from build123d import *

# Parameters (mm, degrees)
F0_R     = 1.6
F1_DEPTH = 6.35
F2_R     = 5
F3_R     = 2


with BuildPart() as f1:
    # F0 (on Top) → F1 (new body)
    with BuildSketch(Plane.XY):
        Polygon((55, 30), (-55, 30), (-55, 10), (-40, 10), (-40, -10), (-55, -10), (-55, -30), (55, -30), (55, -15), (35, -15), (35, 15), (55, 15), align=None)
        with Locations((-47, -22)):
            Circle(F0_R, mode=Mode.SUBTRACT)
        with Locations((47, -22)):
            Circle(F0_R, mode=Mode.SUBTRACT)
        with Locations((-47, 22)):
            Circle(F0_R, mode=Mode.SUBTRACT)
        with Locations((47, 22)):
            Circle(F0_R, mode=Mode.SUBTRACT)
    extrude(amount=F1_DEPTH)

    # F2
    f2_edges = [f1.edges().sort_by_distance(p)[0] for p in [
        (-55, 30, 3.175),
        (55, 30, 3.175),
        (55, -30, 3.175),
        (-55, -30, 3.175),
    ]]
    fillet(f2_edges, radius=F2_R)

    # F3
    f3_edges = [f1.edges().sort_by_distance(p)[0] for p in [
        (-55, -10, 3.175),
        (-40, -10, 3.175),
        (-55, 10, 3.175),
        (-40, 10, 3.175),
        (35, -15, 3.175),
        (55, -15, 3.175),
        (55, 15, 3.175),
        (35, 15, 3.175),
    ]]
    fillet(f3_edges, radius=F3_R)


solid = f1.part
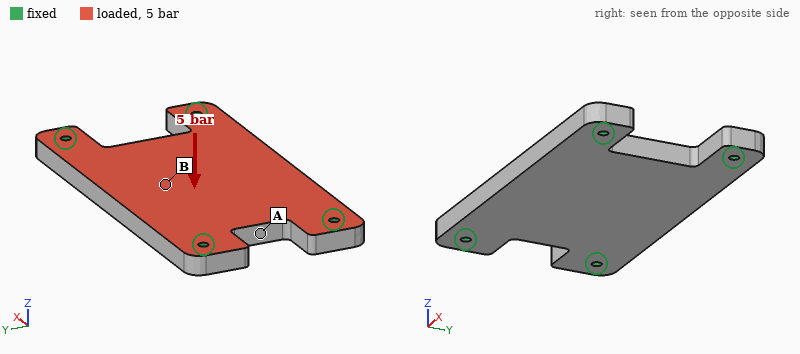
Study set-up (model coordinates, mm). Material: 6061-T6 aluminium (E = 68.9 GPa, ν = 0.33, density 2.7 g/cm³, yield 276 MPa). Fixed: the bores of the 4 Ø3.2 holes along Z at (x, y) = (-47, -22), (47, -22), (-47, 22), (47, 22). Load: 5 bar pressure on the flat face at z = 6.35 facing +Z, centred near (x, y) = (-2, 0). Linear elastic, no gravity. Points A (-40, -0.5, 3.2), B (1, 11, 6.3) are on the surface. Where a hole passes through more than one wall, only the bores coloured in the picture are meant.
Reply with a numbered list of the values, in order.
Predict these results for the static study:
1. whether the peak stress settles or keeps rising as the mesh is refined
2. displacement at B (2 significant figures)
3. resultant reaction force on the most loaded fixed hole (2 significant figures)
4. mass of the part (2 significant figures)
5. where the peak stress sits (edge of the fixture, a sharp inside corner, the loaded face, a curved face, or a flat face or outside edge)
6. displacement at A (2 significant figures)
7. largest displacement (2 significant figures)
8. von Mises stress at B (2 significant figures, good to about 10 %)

1. keeps rising
2. 0.10 mm
3. 750 N
4. 97 g
5. edge of the fixture
6. 0.020 mm
7. 0.11 mm
8. 31 MPa
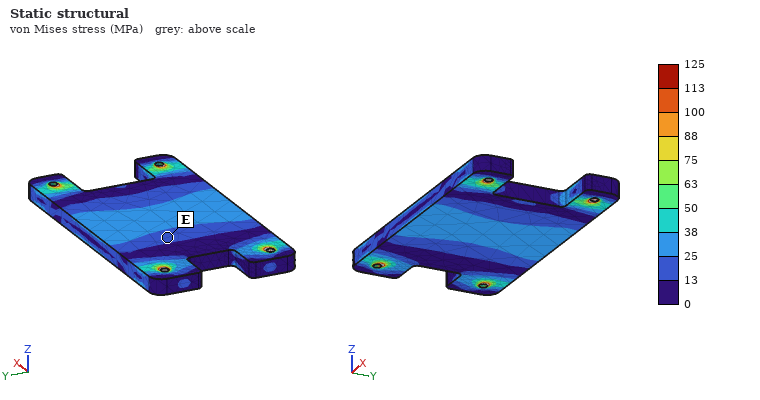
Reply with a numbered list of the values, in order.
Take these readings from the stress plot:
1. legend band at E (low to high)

1. 13 to 25 MPa
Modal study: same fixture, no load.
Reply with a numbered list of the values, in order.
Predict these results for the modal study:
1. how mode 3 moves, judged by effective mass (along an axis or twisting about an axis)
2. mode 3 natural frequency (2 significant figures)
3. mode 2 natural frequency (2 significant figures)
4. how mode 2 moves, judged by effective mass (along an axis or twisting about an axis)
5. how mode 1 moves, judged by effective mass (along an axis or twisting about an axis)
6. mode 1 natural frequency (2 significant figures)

1. twisting about Y
2. 8100 Hz
3. 4700 Hz
4. twisting about X
5. along Z
6. 3000 Hz
